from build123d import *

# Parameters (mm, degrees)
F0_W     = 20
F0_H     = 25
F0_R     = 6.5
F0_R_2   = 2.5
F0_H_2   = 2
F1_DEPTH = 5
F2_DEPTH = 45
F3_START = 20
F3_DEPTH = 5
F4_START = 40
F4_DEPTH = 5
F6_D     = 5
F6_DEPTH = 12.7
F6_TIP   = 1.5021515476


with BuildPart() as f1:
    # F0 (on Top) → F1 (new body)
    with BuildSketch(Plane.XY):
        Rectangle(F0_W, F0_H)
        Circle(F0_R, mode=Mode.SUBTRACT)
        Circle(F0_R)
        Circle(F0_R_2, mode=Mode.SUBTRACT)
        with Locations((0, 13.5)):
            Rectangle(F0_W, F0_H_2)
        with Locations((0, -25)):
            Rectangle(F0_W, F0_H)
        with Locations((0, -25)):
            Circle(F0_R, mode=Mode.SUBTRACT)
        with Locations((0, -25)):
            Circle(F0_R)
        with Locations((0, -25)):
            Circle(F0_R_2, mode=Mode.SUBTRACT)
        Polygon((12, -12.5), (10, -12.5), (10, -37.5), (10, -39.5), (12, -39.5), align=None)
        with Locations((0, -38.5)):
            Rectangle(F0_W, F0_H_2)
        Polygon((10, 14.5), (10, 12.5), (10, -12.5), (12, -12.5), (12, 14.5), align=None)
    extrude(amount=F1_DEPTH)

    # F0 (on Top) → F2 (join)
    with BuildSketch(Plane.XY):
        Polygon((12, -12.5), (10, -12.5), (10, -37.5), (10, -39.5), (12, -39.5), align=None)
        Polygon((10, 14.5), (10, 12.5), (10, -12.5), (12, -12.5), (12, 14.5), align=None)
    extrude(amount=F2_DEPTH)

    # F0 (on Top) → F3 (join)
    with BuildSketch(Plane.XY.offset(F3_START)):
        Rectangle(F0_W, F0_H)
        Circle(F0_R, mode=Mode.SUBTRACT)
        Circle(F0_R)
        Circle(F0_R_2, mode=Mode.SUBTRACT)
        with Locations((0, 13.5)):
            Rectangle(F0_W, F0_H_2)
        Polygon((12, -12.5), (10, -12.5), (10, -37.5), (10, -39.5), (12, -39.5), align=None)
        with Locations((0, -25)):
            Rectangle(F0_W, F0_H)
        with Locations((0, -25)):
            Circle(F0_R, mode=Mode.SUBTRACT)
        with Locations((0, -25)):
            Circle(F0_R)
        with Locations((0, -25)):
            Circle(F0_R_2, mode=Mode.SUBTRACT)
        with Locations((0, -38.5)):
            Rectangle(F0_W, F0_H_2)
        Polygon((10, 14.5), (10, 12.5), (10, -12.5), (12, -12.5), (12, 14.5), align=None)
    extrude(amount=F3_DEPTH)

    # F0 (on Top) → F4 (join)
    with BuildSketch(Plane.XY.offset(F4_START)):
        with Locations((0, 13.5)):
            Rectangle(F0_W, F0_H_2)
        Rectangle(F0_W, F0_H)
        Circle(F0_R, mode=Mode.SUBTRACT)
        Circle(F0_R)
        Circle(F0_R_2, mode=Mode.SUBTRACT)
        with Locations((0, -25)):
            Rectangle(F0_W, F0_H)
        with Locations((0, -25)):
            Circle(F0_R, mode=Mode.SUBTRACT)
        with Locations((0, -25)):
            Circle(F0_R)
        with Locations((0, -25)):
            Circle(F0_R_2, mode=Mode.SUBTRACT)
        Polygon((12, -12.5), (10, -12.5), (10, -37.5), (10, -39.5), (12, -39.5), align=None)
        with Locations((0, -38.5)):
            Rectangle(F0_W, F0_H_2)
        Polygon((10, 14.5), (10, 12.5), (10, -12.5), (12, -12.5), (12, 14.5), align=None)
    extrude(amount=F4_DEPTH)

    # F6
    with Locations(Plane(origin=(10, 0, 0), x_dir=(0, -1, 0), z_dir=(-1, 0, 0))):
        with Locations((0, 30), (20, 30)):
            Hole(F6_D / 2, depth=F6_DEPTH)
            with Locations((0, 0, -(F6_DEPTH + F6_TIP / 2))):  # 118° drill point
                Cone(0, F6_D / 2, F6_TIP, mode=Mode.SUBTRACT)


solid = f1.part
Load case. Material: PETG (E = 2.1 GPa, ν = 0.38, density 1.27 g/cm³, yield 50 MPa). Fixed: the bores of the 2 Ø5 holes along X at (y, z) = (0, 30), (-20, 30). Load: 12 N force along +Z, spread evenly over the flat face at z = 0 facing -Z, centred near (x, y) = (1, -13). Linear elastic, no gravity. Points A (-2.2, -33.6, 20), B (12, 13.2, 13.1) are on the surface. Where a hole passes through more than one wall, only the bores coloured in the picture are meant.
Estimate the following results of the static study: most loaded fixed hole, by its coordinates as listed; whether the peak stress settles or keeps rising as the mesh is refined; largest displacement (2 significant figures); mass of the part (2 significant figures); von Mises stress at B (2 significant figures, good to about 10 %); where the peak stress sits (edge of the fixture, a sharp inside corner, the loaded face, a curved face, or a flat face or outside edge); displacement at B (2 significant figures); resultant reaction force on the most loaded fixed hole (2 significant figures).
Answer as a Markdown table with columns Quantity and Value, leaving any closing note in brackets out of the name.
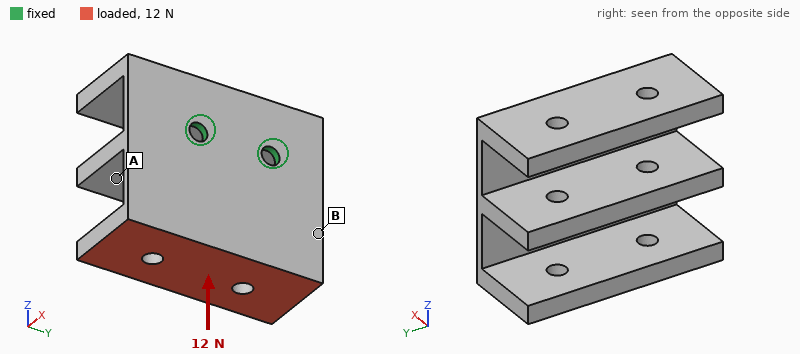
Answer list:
| Quantity | Value |
|---|---|
| most loaded fixed hole, by its coordinates as listed | (-20, 30) |
| whether the peak stress settles or keeps rising as the mesh is refined | keeps rising |
| largest displacement | 0.83 mm |
| mass of the part | 26 g |
| von Mises stress at B | 3.2 MPa |
| where the peak stress sits | edge of the fixture |
| displacement at B | 0.14 mm |
| resultant reaction force on the most loaded fixed hole | 7.3 N |
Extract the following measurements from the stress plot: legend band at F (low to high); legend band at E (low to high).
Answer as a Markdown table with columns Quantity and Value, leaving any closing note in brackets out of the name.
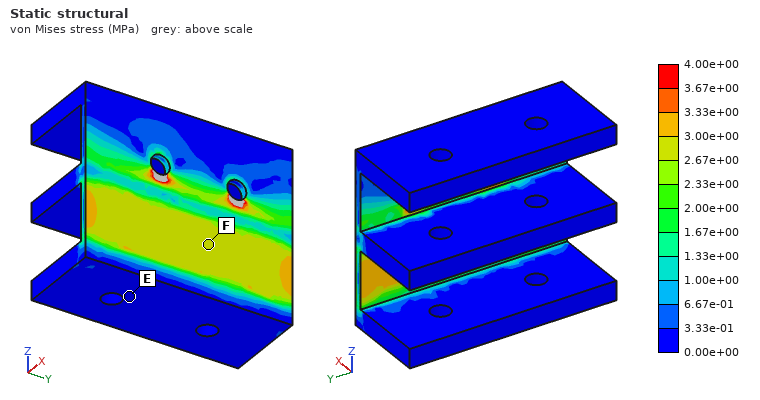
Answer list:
| Quantity | Value |
|---|---|
| legend band at F | 2.67e+00 to 3.00e+00 MPa |
| legend band at E | 0.00e+00 to 3.33e-01 MPa |
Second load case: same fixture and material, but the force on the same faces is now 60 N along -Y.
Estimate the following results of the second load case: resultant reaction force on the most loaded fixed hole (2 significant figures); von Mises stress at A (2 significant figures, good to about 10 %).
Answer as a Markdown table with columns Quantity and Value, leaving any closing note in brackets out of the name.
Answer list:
| Quantity | Value |
|---|---|
| resultant reaction force on the most loaded fixed hole | 87 N |
| von Mises stress at A | 1.2 MPa |
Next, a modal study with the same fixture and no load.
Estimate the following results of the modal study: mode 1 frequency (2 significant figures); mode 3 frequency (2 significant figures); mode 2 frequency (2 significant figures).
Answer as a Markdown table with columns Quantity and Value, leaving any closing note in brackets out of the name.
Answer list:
| Quantity | Value |
|---|---|
| mode 1 frequency | 180 Hz |
| mode 3 frequency | 490 Hz |
| mode 2 frequency | 380 Hz |
